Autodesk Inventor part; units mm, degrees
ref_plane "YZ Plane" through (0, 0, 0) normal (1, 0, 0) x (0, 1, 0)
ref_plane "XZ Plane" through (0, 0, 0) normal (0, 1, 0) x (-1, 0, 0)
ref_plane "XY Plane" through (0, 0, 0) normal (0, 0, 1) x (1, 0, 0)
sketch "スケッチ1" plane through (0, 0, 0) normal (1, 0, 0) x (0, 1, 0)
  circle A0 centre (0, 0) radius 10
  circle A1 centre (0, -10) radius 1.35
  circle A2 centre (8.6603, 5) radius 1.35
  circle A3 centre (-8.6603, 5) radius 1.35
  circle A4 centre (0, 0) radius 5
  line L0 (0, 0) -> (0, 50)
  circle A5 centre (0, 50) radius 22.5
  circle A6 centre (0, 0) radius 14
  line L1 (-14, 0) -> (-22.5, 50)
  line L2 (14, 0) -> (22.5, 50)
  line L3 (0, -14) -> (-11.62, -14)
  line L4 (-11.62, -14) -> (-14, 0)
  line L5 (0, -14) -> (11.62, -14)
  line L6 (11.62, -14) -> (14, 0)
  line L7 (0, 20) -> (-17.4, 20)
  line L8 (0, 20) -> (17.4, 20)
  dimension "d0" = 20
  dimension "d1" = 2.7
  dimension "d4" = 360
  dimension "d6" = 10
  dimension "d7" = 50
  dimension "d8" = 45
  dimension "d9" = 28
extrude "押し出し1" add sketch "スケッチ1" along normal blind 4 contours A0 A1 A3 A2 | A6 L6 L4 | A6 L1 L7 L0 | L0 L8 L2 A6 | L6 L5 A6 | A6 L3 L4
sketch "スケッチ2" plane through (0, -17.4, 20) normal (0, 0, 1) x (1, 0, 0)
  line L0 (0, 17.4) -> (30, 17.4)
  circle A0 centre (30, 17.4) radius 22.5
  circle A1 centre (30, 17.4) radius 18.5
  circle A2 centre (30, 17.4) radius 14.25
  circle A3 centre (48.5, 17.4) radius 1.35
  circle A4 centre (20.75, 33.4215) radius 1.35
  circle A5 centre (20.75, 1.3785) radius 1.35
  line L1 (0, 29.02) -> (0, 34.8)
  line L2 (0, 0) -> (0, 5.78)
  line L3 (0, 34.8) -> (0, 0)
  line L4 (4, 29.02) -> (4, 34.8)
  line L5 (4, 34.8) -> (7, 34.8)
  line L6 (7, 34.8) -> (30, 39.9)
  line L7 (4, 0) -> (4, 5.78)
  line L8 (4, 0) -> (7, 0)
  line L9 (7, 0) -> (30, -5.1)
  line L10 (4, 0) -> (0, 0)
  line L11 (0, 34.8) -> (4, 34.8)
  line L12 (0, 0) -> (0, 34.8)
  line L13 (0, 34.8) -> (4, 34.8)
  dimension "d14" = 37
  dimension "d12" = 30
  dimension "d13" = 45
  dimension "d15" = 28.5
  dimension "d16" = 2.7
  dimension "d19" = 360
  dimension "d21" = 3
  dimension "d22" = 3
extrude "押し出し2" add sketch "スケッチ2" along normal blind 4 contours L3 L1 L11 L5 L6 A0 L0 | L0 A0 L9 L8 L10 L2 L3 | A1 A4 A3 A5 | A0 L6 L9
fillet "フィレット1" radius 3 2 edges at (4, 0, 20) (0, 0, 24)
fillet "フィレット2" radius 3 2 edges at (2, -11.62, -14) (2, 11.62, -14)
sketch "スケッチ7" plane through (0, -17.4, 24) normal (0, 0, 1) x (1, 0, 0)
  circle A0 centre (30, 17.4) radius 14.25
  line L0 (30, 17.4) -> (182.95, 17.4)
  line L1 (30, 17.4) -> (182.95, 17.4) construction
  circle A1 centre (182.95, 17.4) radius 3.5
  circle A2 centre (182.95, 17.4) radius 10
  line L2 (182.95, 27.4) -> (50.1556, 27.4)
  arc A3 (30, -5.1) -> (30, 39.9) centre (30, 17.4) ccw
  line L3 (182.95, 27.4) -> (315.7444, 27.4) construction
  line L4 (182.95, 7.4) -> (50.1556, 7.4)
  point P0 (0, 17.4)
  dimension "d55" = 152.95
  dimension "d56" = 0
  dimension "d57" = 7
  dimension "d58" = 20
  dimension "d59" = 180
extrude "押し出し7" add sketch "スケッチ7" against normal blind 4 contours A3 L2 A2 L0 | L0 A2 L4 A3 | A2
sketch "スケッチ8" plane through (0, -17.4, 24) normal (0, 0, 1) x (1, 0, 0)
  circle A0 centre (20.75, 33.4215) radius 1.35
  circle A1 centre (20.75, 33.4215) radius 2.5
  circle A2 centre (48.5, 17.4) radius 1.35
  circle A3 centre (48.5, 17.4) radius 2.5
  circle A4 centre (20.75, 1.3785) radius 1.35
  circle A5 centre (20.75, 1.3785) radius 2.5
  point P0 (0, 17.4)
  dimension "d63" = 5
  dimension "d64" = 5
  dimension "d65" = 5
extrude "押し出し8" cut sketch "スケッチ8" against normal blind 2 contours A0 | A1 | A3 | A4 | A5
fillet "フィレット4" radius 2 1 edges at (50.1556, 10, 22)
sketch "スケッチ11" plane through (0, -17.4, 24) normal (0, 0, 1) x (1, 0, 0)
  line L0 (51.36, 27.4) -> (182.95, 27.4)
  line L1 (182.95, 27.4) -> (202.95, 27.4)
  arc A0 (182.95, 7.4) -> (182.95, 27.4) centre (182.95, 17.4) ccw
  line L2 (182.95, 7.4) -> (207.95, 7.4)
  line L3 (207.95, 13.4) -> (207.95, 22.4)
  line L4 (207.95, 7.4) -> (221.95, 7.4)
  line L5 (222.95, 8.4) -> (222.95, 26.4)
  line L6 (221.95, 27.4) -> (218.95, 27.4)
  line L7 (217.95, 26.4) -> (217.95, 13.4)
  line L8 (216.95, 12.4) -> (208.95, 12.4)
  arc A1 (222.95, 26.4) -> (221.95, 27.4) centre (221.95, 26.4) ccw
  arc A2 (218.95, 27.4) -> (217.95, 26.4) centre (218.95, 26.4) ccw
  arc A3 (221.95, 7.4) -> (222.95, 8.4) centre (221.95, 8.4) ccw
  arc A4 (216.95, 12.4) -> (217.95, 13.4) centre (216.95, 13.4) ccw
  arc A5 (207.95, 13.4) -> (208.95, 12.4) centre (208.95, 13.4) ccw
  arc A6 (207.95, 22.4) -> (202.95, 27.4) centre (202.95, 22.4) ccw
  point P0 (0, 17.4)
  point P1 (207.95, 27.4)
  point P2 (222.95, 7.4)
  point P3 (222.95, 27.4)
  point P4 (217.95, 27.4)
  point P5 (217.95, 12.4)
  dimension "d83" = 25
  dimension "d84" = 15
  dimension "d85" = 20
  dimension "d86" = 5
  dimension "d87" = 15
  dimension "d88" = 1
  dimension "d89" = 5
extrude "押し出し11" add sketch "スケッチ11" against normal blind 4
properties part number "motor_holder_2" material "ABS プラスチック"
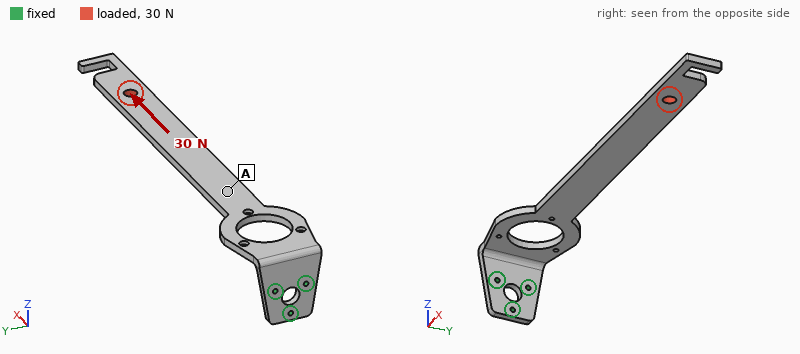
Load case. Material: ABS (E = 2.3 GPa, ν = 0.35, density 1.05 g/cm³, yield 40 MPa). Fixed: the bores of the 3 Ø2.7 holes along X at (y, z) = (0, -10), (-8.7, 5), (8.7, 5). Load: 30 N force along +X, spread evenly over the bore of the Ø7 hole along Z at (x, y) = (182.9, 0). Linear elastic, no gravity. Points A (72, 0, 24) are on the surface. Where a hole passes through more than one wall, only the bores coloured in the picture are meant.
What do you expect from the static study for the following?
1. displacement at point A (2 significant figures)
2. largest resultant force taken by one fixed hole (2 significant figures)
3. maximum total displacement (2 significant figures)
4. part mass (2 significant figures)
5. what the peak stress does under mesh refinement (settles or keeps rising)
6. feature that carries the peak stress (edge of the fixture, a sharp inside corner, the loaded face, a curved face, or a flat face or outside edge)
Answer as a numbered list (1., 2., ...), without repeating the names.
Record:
1. 0.87 mm
2. 17 N
3. 2.7 mm
4. 23 g
5. keeps rising
6. edge of the fixture
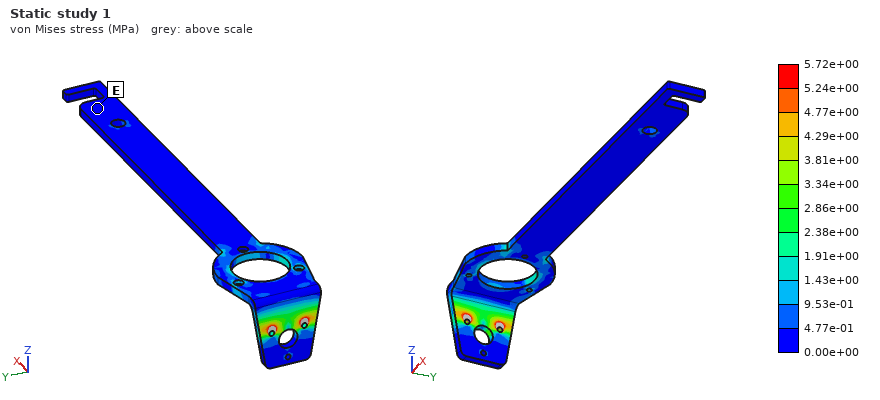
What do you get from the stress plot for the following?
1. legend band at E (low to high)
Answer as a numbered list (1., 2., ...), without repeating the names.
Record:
1. 0.00e+00 to 4.77e-01 MPa
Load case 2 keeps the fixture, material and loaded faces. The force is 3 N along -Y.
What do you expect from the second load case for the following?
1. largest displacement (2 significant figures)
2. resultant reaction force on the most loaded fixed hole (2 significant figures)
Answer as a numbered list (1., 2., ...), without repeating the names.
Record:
1. 2.4 mm
2. 26 N
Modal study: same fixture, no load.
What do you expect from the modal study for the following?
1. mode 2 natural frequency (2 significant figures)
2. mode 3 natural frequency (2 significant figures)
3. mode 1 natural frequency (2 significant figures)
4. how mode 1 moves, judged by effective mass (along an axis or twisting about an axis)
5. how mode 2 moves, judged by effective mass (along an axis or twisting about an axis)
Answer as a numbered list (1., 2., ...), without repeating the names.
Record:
1. 72 Hz
2. 120 Hz
3. 19 Hz
4. along Z
5. along Y
